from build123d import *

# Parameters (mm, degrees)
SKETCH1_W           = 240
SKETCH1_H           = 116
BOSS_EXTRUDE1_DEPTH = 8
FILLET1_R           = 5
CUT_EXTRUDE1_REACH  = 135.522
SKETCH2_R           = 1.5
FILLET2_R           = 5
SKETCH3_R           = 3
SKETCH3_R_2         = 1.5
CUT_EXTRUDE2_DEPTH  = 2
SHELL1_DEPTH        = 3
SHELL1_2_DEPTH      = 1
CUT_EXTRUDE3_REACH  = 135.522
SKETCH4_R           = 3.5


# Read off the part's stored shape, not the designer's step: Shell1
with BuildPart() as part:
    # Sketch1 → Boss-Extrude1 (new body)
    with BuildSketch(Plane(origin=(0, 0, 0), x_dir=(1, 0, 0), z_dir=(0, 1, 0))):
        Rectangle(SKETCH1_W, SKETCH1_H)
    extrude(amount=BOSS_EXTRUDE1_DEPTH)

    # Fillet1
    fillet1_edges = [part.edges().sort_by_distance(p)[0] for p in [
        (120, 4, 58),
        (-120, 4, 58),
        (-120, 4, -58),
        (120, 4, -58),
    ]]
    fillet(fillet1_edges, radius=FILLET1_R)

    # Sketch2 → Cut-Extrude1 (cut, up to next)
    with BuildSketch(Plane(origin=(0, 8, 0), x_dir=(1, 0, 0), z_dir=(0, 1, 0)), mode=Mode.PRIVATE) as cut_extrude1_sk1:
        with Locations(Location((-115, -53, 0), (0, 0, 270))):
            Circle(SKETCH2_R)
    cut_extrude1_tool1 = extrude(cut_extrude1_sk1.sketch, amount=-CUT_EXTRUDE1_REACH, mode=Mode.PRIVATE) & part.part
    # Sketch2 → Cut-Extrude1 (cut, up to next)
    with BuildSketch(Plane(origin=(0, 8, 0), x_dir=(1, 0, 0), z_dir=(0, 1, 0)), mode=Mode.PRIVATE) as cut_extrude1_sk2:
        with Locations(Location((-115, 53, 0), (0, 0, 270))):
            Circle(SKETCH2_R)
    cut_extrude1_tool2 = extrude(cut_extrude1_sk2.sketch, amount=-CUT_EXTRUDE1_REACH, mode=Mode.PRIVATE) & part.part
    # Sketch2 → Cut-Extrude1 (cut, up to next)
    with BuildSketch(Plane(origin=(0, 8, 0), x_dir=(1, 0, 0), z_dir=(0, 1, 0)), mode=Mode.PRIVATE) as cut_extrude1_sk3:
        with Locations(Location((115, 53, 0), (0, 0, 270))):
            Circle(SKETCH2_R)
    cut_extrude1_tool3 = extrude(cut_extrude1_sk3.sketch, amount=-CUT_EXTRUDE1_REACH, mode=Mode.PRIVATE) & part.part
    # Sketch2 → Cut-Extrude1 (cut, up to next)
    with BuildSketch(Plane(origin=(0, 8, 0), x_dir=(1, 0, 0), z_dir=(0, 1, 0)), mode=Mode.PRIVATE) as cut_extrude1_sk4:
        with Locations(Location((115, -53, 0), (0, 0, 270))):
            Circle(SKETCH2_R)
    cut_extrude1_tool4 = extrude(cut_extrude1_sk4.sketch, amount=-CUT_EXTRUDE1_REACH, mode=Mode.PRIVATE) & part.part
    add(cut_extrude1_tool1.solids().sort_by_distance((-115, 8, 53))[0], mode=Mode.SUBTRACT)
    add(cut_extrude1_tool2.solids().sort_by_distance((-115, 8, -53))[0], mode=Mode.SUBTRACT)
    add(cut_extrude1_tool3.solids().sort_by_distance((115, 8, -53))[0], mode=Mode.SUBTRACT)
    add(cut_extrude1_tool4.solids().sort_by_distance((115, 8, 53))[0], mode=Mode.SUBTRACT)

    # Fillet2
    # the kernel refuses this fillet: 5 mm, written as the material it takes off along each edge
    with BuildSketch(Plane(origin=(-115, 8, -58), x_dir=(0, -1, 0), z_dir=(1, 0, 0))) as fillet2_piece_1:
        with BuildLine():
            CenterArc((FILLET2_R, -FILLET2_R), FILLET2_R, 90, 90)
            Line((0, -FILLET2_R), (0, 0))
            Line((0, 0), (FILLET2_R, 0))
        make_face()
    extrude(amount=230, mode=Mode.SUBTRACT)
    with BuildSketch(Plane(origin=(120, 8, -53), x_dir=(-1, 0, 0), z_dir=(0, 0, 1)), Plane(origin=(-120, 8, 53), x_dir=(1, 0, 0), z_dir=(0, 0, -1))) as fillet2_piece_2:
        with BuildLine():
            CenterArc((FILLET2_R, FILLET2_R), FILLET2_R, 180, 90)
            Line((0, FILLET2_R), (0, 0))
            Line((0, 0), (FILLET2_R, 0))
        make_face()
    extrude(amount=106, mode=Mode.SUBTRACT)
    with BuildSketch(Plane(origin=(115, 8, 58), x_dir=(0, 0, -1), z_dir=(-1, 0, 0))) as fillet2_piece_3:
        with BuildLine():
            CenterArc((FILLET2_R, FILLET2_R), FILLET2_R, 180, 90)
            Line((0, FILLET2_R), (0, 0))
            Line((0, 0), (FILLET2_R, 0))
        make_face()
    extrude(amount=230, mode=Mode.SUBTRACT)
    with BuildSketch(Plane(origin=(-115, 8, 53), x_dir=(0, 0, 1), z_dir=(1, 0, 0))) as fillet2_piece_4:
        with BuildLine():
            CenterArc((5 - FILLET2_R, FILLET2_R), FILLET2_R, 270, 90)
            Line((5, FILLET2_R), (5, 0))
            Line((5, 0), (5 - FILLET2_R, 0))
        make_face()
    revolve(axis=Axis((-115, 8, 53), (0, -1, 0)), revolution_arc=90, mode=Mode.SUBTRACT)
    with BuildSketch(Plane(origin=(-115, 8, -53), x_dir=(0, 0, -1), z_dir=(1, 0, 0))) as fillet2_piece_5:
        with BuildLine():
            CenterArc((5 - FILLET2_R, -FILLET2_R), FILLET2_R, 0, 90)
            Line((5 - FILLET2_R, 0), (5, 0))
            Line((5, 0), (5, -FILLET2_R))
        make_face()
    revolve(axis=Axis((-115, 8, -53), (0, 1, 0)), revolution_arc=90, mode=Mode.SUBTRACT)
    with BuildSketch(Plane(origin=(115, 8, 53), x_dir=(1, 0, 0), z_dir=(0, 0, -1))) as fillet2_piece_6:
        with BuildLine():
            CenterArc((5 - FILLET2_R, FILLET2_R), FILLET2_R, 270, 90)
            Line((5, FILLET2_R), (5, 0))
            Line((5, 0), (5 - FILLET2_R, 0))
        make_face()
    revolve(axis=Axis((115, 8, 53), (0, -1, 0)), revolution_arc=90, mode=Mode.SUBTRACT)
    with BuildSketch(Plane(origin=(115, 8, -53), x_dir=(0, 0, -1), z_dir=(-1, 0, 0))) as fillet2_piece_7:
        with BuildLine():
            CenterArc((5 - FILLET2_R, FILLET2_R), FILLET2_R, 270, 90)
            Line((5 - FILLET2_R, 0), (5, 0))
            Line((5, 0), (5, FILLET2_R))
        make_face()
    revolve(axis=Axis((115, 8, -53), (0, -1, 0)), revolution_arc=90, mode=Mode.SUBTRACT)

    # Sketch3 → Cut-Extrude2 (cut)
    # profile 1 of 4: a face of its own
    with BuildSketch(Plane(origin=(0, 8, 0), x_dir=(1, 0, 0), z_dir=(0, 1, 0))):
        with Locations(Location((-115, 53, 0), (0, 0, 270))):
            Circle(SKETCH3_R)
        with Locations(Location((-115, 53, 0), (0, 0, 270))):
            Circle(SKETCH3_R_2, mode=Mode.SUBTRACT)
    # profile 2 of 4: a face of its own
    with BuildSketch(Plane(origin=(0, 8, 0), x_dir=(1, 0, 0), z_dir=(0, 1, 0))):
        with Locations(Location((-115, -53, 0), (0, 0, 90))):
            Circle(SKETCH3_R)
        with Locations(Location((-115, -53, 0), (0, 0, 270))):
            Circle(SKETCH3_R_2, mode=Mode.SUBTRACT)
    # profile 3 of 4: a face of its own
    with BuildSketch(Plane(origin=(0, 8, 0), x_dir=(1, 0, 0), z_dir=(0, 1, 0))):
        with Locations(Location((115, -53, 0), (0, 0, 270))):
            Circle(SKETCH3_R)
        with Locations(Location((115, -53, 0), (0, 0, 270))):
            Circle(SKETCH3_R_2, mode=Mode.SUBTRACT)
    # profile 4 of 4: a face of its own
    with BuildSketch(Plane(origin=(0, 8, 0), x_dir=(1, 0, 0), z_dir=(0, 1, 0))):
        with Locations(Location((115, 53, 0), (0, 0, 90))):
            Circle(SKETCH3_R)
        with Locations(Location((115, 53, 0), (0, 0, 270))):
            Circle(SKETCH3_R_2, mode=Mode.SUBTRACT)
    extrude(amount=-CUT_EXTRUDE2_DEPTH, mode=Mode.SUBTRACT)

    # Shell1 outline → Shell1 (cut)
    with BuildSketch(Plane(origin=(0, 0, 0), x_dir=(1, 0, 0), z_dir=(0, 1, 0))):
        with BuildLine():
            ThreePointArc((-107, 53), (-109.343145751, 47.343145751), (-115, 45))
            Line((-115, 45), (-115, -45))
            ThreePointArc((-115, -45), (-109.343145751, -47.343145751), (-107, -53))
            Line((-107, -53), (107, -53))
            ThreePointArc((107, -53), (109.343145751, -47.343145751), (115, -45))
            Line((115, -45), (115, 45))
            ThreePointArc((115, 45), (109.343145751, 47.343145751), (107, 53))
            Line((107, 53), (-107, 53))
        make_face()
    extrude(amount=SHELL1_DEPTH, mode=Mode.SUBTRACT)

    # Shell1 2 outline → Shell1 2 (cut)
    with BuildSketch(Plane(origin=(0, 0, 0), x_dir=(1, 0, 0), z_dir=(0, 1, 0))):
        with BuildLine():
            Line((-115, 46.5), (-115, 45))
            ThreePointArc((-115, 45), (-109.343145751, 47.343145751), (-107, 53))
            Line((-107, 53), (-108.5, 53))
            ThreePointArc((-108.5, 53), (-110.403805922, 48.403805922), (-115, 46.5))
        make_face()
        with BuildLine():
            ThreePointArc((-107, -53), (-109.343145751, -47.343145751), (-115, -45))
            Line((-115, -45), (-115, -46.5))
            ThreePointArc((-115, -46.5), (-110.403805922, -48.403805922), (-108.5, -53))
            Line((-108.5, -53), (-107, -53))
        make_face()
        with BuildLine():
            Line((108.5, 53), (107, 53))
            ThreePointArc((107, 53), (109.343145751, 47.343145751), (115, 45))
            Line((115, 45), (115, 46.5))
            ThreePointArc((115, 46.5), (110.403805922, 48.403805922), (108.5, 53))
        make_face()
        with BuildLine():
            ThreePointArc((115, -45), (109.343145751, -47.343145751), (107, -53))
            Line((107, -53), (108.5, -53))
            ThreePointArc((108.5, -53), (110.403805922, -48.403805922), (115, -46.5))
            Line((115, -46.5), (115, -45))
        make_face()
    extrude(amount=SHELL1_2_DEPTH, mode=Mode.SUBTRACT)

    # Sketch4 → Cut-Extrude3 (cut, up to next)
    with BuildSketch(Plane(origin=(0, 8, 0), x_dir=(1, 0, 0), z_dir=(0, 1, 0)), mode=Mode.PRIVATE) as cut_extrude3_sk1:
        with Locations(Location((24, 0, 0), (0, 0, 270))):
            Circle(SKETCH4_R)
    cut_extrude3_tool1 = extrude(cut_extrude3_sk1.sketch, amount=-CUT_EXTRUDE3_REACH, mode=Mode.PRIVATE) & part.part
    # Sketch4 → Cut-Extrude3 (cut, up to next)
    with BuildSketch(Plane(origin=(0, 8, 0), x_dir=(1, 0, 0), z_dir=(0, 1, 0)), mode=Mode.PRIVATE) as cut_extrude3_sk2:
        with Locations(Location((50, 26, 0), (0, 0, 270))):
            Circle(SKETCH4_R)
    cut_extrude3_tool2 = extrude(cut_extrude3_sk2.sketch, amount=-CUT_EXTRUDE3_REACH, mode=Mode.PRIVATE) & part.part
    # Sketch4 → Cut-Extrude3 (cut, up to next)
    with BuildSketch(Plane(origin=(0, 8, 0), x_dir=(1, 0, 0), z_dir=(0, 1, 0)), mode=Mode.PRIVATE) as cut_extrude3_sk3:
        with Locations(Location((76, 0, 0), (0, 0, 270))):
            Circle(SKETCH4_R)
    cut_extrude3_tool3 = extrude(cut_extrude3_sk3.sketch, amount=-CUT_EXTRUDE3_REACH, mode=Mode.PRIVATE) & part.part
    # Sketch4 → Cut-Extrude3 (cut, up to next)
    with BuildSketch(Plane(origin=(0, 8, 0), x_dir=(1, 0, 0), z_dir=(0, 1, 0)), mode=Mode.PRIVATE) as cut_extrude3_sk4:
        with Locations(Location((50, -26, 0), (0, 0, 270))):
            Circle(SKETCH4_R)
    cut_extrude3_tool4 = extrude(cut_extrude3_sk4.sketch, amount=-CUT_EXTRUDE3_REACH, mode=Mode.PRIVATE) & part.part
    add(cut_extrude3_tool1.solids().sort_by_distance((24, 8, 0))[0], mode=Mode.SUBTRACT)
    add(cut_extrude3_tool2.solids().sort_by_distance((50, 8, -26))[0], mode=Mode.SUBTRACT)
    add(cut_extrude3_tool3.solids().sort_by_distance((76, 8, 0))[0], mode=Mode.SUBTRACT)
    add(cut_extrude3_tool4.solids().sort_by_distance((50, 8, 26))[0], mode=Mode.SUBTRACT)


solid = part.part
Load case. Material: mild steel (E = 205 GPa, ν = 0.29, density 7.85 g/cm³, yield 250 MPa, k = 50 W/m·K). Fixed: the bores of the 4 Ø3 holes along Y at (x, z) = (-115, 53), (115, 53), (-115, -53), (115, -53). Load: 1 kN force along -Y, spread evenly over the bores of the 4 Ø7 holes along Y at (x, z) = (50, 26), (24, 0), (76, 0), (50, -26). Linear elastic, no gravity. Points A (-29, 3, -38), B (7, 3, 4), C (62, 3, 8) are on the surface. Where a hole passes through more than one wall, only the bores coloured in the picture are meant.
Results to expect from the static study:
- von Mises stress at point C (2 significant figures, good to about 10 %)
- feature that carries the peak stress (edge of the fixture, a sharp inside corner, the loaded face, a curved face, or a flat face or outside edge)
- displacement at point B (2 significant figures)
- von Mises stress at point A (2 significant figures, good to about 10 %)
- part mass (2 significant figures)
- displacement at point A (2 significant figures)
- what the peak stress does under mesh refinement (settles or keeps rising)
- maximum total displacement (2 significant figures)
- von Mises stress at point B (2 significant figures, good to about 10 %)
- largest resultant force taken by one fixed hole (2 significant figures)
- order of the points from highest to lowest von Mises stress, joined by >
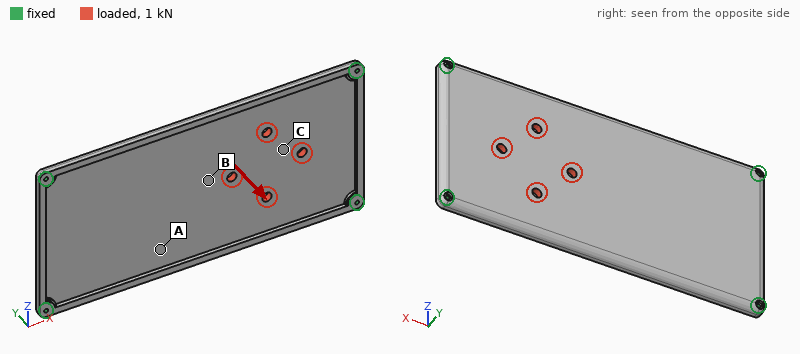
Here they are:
23 MPa
edge of the fixture
0.18 mm
7.0 MPa
1.1 kg
0.13 mm
keeps rising
0.19 mm
19 MPa
860 N
C > B > A
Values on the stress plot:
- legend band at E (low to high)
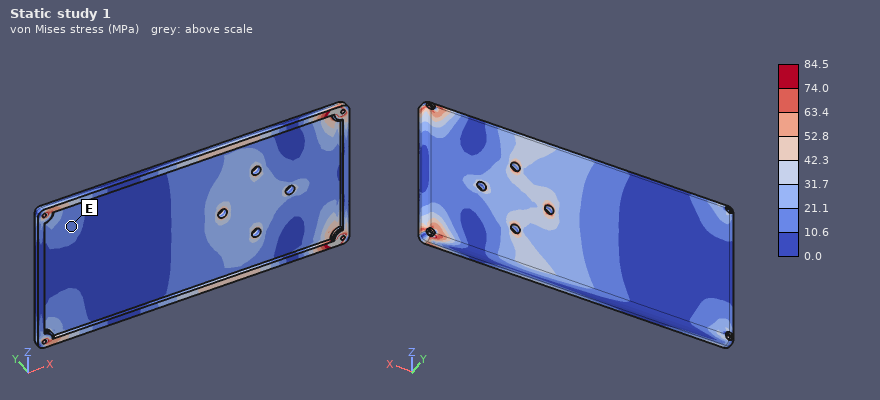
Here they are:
10.6 to 21.1 MPa
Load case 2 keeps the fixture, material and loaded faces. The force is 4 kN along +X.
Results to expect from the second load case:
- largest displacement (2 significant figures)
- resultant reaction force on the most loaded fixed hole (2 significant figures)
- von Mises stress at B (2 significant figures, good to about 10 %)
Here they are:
7.1 µm
1.3 kN
5.3 MPa
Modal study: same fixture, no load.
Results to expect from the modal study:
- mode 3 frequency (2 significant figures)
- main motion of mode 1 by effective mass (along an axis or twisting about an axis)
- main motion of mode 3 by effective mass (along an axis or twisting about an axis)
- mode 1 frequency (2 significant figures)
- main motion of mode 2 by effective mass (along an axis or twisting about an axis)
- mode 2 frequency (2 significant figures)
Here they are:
1300 Hz
along Y
twisting about Z
470 Hz
twisting about X
860 Hz
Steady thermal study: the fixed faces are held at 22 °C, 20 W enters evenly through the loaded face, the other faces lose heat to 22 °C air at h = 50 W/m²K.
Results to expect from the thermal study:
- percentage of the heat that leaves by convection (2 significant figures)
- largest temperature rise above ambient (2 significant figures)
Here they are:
83 %
17 K
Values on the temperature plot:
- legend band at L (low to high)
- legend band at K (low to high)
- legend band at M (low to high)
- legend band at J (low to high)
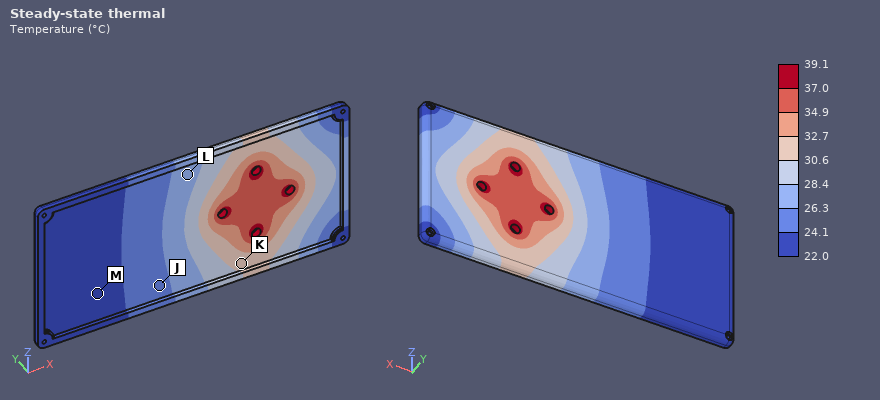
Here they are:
26.3 to 28.4 °C
30.6 to 32.7 °C
22.0 to 24.1 °C
24.1 to 26.3 °C
